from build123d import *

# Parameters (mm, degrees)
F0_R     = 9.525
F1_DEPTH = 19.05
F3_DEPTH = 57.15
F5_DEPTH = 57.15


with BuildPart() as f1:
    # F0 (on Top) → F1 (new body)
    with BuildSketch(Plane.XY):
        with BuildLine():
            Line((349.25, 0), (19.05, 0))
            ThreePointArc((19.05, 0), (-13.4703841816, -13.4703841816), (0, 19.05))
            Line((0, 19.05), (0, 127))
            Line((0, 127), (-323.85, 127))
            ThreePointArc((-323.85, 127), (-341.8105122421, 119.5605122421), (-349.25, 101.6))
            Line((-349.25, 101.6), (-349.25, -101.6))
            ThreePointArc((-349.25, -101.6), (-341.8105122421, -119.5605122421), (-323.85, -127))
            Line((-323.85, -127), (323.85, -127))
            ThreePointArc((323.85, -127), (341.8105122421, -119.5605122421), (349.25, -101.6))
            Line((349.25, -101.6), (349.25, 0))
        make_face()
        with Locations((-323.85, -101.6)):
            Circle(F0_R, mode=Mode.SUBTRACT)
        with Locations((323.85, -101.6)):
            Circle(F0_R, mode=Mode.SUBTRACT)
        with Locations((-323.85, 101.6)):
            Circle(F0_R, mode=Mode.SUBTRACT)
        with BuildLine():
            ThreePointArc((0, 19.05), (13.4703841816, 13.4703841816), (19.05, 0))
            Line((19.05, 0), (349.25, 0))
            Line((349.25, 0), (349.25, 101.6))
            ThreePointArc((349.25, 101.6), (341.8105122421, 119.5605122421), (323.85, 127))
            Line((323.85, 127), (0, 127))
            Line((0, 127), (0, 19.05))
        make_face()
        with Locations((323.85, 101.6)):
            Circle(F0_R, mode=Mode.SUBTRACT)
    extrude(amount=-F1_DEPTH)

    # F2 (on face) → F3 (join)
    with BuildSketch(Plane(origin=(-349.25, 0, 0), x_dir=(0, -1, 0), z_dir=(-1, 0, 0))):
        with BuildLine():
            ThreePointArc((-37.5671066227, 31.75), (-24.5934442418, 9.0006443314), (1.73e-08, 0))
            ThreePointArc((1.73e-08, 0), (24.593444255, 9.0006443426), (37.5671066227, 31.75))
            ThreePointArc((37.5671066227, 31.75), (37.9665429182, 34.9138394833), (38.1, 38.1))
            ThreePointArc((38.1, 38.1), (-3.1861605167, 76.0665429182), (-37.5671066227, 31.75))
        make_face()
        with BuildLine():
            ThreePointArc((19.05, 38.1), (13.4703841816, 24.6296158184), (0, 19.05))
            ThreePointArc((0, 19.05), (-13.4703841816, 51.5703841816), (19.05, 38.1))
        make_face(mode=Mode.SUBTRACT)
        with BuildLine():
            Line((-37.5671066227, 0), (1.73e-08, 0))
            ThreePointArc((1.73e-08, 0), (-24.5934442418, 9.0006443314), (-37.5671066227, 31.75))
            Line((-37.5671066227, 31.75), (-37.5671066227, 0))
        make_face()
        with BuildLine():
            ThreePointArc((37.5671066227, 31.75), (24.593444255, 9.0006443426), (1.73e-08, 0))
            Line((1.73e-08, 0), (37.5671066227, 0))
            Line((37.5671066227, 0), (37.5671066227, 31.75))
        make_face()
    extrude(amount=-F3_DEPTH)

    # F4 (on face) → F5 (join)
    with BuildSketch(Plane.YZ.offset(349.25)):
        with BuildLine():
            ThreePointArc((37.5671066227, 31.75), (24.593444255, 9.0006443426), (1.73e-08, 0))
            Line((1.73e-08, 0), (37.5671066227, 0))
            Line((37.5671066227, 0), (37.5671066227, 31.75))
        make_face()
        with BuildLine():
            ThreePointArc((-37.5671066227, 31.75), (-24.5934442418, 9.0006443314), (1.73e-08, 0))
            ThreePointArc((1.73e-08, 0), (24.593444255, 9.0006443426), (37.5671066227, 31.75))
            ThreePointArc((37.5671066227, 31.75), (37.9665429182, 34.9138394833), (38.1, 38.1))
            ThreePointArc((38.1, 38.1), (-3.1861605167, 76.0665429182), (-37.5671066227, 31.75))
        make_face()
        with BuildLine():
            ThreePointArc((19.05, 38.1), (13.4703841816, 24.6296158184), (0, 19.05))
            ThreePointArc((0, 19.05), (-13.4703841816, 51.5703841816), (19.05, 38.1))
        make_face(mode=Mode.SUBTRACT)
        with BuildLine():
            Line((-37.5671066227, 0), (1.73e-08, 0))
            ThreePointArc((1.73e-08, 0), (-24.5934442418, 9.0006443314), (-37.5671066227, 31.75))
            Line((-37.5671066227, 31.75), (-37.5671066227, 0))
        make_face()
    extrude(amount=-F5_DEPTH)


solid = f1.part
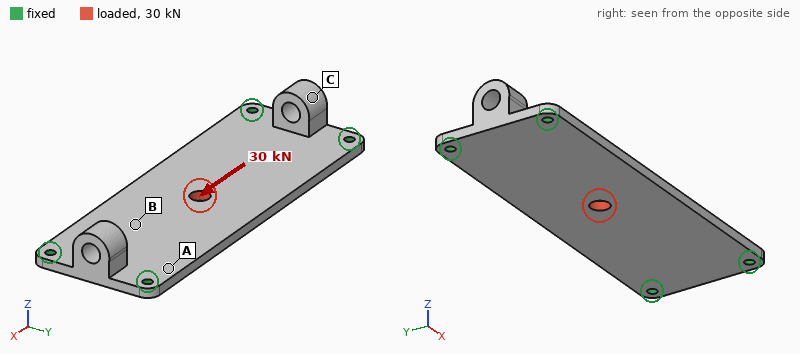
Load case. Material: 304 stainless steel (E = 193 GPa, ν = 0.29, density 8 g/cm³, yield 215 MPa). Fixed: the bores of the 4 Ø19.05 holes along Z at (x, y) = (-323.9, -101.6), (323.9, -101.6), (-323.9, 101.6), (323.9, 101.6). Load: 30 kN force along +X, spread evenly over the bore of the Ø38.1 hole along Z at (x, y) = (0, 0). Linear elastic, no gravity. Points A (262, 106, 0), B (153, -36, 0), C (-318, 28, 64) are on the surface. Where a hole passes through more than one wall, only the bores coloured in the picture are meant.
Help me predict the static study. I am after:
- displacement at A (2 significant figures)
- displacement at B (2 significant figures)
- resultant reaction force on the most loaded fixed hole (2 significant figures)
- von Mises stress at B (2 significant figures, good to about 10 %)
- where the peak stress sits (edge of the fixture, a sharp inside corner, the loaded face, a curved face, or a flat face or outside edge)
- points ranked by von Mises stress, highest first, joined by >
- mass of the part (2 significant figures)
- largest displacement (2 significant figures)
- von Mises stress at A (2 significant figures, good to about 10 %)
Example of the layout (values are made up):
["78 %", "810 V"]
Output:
["1.8 µm", "4.1 µm", "7.7 kN", "3.6 MPa", "the loaded face", "A > B > C", "30 kg", "8.9 µm", "4.8 MPa"]
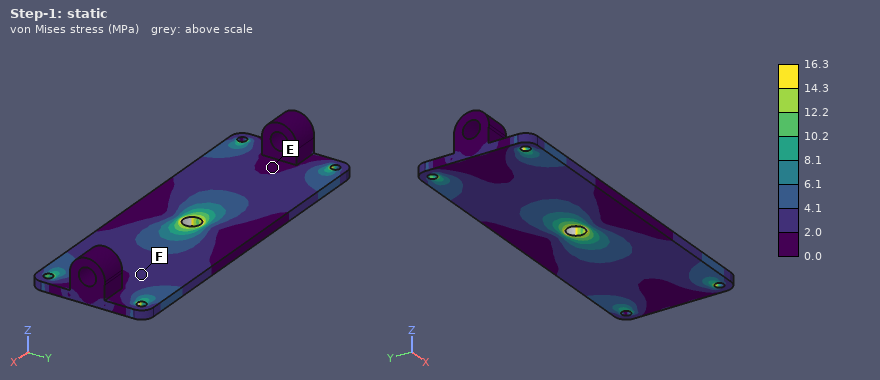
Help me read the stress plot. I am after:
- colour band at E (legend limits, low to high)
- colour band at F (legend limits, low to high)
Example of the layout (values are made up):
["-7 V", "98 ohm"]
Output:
["0.0 to 2.0 MPa", "2.0 to 4.1 MPa"]
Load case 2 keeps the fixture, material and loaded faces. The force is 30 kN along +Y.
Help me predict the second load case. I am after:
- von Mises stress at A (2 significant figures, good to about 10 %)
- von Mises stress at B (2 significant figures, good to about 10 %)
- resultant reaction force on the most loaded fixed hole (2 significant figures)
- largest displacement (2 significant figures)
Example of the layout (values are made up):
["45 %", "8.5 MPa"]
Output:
["7.0 MPa", "7.3 MPa", "14 kN", "26 µm"]
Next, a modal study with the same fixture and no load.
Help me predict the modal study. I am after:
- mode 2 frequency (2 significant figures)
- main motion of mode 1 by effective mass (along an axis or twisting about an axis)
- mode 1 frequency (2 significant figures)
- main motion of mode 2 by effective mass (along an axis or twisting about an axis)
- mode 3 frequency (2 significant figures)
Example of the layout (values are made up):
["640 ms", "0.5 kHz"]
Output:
["450 Hz", "along Z", "210 Hz", "twisting about X", "580 Hz"]
